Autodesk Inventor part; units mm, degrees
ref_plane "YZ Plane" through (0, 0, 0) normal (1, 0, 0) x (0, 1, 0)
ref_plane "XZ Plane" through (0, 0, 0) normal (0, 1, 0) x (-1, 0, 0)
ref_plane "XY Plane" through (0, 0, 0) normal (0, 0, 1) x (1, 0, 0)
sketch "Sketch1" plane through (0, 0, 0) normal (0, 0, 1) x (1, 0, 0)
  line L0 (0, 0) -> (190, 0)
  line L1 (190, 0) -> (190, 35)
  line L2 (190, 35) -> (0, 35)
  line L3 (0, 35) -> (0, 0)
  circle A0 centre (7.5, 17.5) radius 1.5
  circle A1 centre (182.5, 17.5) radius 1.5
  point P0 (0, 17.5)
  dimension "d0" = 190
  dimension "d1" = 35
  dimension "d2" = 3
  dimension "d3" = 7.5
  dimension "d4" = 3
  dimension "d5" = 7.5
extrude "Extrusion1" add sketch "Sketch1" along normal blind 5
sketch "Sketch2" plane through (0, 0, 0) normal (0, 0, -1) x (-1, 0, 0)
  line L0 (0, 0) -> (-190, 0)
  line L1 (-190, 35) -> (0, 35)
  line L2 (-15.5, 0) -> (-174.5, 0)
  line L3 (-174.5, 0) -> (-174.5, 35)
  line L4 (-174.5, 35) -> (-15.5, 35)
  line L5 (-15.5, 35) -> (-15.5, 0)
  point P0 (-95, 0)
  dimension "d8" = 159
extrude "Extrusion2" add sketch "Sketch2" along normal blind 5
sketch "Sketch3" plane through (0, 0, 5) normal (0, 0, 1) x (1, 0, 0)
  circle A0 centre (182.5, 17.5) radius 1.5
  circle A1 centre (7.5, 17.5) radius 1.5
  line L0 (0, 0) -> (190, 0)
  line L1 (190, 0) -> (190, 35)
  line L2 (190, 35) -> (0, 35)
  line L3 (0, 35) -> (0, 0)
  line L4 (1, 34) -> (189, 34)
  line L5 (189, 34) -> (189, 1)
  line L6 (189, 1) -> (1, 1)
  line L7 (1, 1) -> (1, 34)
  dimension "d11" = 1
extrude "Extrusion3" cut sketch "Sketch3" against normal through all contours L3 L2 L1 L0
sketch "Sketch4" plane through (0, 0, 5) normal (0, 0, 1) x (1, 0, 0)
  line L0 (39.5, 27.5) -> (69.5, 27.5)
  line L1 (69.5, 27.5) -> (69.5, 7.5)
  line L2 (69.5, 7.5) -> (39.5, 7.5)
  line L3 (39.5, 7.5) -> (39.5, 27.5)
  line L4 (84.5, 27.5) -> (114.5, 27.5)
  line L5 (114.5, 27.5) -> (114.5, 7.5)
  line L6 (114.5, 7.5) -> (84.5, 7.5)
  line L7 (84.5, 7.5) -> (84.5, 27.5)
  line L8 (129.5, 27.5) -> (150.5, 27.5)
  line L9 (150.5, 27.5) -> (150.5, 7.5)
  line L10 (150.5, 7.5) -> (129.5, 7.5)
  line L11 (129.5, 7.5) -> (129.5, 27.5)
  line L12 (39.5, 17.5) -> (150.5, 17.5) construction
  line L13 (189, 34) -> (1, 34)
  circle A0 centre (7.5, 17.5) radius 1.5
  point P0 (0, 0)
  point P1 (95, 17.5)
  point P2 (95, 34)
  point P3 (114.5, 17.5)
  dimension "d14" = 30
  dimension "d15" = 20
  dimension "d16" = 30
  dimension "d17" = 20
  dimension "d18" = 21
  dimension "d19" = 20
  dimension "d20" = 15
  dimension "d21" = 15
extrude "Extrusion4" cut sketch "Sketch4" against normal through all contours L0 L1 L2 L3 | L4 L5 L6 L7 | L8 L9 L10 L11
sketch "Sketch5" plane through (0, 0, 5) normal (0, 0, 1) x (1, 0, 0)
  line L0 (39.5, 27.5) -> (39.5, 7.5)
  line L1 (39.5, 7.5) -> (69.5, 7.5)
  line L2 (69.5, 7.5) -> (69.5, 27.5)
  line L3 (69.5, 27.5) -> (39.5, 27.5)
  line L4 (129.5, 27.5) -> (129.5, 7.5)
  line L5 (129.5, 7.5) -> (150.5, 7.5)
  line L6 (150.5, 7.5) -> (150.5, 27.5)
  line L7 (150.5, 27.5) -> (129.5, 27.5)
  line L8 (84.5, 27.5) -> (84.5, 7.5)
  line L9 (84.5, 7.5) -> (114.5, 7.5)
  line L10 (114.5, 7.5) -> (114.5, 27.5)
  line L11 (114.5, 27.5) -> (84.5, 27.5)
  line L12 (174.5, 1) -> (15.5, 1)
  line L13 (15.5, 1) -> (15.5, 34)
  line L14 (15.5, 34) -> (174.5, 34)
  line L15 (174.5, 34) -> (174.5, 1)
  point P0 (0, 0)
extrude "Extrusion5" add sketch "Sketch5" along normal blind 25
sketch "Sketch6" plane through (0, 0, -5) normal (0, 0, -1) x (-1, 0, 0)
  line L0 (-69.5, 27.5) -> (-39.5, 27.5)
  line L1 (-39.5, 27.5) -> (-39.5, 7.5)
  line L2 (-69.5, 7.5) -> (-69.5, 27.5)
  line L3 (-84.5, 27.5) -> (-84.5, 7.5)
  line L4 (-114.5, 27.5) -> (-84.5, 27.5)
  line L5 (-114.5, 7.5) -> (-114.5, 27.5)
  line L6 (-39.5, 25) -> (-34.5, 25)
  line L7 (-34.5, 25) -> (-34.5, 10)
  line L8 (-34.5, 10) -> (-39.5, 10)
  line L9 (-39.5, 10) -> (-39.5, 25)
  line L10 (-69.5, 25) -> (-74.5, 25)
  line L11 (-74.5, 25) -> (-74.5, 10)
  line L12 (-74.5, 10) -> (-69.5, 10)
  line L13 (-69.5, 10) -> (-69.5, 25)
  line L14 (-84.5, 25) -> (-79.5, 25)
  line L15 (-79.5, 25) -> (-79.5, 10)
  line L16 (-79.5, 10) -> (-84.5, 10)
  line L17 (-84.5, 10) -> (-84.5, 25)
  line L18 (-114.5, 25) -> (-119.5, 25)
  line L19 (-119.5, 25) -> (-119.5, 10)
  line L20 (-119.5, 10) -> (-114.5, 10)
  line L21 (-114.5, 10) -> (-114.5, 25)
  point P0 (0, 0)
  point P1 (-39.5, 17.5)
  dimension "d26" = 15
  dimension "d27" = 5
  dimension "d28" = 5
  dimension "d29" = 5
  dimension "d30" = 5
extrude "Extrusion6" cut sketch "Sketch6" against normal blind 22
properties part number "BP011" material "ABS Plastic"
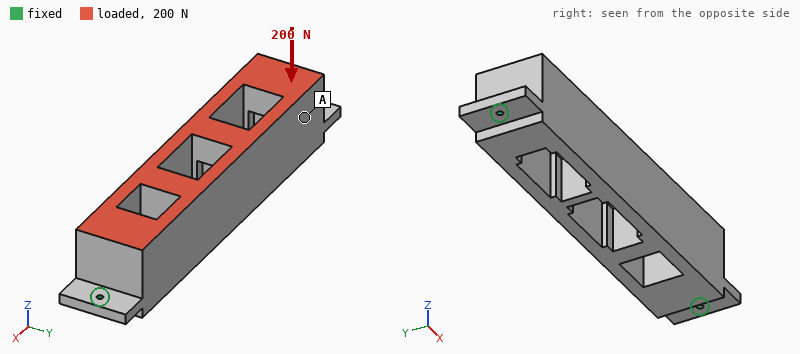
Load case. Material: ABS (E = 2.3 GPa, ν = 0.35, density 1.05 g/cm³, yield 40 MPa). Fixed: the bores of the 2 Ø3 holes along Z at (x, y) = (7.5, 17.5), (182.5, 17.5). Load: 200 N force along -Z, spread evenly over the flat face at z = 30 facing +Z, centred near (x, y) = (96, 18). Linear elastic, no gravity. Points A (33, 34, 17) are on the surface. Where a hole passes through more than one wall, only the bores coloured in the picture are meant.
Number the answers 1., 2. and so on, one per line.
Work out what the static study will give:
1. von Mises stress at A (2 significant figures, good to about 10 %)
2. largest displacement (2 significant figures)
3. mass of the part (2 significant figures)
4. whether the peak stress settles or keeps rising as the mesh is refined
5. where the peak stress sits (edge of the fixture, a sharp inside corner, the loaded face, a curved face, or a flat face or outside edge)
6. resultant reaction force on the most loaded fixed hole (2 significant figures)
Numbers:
1. 0.44 MPa
2. 0.12 mm
3. 130 g
4. keeps rising
5. edge of the fixture
6. 140 N
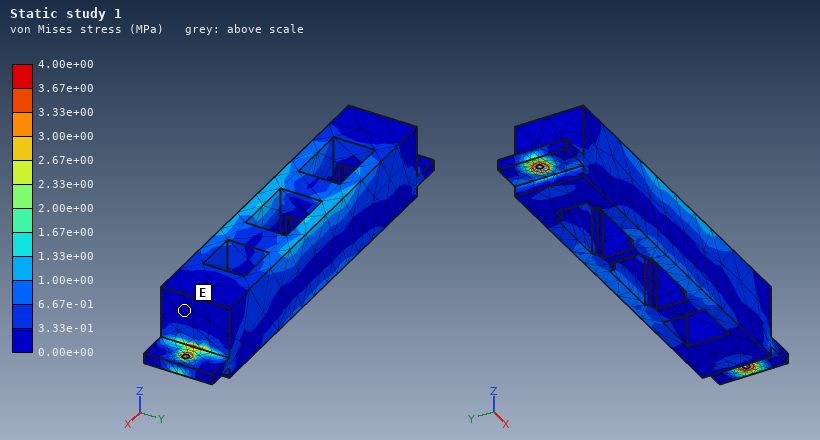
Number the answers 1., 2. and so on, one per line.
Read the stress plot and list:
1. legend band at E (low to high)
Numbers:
1. 0.00e+00 to 3.33e-01 MPa
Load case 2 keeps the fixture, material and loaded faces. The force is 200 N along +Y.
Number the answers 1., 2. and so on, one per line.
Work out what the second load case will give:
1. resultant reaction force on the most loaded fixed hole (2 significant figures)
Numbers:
1. 100 N
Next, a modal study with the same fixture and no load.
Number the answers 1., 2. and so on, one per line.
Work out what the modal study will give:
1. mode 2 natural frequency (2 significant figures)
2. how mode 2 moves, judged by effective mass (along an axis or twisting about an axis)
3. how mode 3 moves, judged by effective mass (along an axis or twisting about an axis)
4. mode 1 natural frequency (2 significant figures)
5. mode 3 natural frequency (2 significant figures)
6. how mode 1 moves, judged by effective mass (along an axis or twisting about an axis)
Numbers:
1. 660 Hz
2. along Z
3. along Y
4. 320 Hz
5. 760 Hz
6. along Y
